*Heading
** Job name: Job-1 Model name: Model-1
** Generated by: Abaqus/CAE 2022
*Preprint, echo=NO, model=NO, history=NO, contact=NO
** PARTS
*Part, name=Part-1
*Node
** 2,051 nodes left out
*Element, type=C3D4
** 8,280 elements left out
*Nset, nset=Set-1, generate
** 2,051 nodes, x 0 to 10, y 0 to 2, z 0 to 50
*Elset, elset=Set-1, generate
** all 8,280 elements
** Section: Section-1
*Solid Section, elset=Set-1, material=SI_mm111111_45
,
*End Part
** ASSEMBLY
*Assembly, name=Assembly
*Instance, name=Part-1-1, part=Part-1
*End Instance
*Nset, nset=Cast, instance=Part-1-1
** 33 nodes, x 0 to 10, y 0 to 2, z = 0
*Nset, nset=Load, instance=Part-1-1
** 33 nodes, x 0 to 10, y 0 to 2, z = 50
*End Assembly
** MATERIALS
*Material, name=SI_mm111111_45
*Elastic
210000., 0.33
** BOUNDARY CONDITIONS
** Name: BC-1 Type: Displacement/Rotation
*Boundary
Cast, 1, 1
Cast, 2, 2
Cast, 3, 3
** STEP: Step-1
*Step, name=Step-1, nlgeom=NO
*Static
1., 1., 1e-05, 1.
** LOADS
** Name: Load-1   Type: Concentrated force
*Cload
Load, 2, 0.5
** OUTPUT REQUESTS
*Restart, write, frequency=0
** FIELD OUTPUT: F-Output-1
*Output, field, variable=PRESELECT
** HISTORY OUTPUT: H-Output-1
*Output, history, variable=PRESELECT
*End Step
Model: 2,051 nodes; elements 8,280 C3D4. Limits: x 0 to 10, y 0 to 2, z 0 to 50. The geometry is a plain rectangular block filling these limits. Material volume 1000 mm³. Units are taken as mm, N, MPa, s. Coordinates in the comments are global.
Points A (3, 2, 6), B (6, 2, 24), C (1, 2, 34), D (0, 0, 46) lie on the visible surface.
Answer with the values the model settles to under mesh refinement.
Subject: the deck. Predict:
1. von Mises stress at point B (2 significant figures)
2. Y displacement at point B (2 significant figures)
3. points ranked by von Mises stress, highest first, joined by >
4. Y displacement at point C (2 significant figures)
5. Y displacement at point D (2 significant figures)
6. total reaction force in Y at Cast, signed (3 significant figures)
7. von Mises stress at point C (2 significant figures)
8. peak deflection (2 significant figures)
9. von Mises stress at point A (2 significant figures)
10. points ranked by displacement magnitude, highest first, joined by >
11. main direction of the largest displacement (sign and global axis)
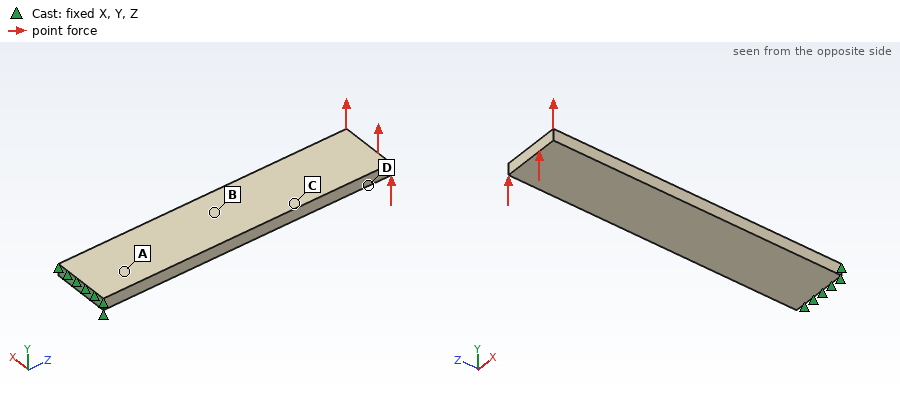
64 MPa
0.14 mm
A > B > C > D
0.26 mm
0.42 mm
-16.5 N
40 MPa
0.48 mm
100 MPa
D > C > B > A
+Y
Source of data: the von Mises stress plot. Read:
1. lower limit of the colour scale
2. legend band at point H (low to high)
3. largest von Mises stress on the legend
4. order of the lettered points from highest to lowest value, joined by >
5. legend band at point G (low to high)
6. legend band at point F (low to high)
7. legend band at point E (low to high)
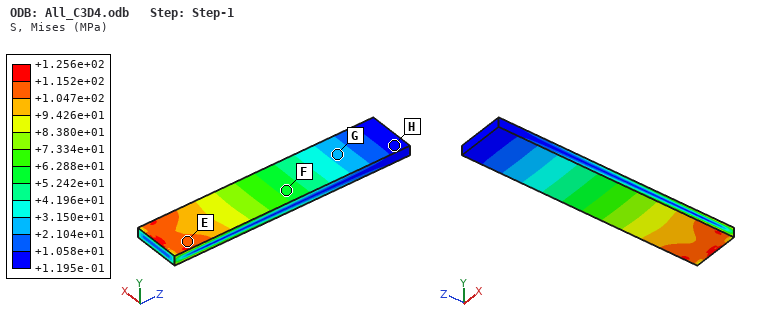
+1.195e-01 MPa
+1.195e-01 to +1.058e+01 MPa
+1.256e+02 MPa
E > F > G > H
+2.104e+01 to +3.150e+01 MPa
+5.242e+01 to +6.288e+01 MPa
+1.047e+02 to +1.152e+02 MPa
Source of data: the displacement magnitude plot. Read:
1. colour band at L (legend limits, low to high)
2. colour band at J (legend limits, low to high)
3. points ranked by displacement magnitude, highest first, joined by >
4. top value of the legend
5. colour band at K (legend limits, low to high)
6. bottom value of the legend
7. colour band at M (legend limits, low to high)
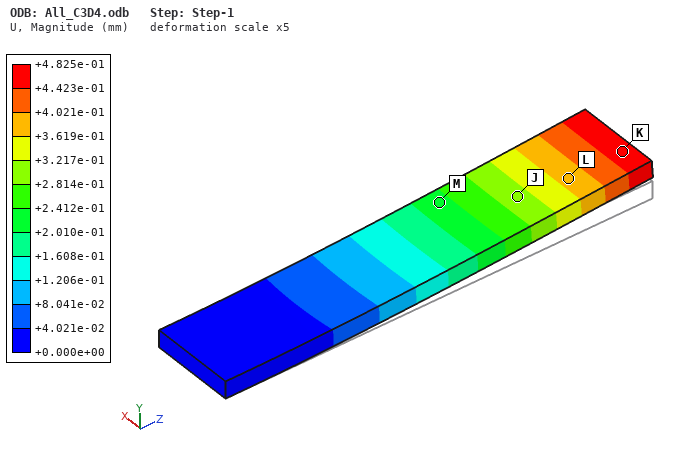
+3.619e-01 to +4.021e-01 mm
+2.814e-01 to +3.217e-01 mm
K > L > J > M
+4.825e-01 mm
+4.423e-01 to +4.825e-01 mm
+0.000e+00 mm
+2.010e-01 to +2.412e-01 mm
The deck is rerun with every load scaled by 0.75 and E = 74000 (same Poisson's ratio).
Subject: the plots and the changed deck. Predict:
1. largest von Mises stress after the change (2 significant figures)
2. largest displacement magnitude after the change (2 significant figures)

94 MPa
1.0 mm
